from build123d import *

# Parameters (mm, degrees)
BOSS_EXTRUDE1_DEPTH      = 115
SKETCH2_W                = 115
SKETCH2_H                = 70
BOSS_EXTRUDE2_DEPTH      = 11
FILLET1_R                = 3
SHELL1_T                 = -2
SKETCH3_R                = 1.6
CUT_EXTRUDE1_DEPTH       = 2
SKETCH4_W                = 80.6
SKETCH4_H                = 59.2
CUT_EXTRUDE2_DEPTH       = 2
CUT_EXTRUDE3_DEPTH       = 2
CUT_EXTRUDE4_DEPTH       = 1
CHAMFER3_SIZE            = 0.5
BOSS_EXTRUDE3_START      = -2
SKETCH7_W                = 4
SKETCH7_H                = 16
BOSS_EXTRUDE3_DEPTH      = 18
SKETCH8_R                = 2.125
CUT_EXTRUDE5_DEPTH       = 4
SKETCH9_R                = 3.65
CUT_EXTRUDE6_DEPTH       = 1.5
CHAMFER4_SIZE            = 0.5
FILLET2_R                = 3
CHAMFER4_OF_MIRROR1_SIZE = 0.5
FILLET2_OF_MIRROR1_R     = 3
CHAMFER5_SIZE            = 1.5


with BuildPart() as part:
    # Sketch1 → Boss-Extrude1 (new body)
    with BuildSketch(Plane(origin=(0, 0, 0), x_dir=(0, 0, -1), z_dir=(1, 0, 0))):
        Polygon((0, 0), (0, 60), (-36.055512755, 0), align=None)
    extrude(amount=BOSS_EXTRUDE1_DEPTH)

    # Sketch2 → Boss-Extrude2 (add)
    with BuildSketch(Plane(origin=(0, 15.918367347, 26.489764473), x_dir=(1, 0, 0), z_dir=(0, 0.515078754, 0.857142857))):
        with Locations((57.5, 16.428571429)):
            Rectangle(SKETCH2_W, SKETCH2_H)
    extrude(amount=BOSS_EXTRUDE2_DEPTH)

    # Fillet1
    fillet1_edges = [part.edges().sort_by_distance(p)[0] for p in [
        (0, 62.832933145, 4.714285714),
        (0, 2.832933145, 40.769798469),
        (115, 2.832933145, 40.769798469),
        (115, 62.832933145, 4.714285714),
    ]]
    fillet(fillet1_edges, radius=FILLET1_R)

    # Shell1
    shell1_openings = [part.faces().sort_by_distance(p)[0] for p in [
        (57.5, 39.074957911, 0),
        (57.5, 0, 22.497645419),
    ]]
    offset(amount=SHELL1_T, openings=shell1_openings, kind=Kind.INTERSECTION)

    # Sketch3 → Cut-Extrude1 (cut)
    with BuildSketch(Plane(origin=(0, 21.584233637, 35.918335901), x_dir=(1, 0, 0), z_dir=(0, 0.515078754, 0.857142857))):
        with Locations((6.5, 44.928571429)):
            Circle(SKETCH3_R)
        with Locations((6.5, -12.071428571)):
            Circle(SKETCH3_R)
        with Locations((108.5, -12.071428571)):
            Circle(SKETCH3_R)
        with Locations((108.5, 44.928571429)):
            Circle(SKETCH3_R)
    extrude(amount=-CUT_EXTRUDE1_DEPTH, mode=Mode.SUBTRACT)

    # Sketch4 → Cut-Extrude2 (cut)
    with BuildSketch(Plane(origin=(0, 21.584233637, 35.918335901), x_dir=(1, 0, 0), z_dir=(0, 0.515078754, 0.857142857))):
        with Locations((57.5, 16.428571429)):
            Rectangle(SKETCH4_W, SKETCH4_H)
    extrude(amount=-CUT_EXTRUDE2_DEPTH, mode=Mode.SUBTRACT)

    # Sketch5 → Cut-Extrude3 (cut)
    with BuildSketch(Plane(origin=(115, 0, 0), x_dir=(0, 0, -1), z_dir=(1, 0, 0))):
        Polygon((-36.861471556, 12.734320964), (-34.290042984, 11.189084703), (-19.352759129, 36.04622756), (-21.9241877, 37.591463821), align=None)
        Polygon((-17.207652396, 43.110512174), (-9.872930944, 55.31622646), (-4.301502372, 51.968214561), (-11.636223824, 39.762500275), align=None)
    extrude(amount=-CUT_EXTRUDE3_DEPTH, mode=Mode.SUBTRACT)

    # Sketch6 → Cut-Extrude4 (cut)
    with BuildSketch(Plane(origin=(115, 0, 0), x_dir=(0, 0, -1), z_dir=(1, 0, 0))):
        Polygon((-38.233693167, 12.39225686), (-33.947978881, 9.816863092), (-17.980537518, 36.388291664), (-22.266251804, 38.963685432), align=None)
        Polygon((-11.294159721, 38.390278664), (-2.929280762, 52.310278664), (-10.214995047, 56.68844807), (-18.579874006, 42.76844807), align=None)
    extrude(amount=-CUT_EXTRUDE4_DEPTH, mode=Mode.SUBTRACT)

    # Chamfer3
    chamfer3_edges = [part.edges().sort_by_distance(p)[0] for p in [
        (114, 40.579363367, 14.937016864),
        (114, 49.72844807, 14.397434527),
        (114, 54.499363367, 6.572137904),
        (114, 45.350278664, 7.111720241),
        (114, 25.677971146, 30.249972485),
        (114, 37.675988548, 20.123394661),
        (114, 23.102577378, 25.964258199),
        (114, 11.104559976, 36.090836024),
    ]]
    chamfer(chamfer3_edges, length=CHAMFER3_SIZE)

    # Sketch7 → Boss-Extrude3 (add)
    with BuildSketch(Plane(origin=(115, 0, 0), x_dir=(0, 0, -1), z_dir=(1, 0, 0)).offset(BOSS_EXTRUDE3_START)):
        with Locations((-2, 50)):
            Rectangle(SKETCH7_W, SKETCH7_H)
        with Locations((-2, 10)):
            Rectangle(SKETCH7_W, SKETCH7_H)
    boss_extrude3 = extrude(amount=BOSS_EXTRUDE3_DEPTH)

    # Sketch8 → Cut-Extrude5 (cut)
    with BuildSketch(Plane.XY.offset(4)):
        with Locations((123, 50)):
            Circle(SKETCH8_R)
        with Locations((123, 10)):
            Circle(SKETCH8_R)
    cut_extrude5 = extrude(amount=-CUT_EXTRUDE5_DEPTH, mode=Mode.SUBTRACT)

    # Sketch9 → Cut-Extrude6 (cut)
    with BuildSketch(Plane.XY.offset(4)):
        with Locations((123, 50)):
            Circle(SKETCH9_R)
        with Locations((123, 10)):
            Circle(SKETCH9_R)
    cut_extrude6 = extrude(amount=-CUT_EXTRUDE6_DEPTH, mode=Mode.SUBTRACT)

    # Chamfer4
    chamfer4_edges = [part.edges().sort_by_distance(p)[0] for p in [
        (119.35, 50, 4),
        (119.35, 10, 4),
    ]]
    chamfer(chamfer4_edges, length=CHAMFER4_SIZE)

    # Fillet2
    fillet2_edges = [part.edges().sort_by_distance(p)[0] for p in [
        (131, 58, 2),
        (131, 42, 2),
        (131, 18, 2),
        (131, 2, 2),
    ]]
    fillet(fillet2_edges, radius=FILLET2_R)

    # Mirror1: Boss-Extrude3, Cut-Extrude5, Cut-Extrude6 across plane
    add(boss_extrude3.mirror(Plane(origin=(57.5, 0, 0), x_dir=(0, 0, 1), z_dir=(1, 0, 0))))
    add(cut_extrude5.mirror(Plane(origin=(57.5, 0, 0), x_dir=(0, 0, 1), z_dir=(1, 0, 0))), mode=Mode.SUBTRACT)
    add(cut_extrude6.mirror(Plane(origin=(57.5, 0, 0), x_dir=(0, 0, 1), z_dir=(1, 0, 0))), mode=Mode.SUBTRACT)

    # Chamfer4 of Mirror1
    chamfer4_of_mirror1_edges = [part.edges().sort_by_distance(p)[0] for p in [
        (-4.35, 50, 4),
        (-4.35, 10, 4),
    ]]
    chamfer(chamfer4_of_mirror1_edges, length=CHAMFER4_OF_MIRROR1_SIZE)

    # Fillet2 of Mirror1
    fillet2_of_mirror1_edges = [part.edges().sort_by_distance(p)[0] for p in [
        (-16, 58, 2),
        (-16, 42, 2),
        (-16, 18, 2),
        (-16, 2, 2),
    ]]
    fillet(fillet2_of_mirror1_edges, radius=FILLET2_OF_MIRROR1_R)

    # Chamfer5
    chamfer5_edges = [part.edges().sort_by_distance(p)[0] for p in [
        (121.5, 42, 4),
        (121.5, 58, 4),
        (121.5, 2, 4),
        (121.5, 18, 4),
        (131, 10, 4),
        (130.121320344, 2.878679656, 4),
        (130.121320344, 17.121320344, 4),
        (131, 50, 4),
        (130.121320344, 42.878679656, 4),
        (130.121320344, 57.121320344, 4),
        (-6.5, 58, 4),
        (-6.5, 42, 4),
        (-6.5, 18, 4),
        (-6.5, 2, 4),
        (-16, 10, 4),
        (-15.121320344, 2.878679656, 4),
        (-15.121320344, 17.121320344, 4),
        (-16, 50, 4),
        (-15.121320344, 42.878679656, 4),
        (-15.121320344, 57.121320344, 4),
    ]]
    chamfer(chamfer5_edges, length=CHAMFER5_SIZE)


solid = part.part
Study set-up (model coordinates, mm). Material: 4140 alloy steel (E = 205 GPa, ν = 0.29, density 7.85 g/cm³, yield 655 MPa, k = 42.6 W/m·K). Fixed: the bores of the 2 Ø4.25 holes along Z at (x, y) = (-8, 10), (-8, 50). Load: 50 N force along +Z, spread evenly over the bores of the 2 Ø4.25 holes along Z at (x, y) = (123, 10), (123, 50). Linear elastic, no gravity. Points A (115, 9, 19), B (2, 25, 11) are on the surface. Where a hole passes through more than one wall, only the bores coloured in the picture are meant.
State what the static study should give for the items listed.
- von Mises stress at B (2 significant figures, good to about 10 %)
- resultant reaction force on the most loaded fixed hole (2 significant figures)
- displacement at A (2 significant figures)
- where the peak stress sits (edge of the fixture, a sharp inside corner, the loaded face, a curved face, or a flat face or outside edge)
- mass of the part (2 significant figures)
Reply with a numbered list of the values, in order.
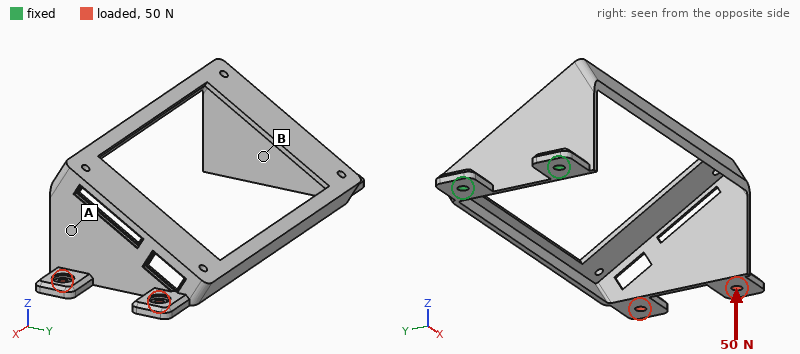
1. 58 MPa
2. 66 N
3. 1.5 mm
4. a curved face
5. 160 g
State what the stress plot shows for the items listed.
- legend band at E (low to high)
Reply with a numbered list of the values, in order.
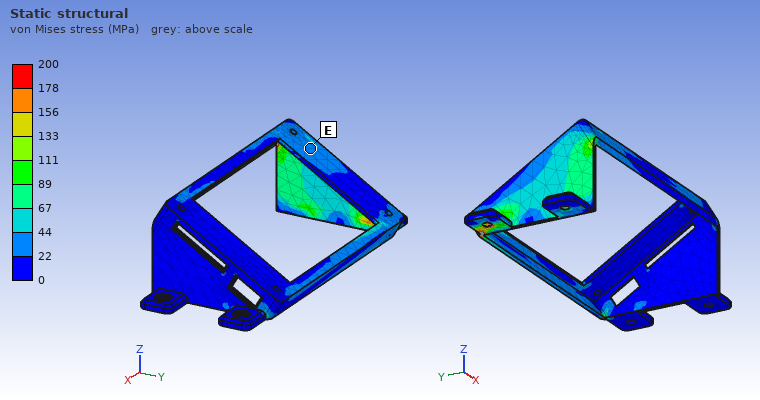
1. 22 to 44 MPa
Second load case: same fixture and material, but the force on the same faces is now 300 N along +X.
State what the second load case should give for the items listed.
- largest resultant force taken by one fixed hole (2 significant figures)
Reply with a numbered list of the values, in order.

1. 160 N
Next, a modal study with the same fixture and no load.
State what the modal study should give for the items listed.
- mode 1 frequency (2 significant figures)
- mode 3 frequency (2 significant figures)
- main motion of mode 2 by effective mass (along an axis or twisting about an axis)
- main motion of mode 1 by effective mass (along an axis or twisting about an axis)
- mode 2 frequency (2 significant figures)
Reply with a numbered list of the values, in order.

1. 110 Hz
2. 380 Hz
3. along Y
4. along Z
5. 170 Hz
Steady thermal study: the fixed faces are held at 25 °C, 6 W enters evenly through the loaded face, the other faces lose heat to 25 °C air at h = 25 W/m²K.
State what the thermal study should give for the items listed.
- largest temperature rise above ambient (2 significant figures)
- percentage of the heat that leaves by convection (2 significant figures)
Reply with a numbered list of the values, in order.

1. 52 K
2. 99 %
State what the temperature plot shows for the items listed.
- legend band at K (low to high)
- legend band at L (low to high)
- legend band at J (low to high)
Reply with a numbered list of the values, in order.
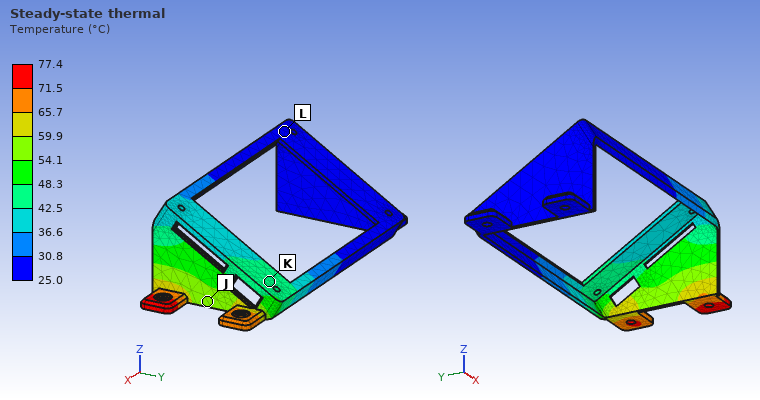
1. 42.5 to 48.3 °C
2. 25.0 to 30.8 °C
3. 54.1 to 59.9 °C
